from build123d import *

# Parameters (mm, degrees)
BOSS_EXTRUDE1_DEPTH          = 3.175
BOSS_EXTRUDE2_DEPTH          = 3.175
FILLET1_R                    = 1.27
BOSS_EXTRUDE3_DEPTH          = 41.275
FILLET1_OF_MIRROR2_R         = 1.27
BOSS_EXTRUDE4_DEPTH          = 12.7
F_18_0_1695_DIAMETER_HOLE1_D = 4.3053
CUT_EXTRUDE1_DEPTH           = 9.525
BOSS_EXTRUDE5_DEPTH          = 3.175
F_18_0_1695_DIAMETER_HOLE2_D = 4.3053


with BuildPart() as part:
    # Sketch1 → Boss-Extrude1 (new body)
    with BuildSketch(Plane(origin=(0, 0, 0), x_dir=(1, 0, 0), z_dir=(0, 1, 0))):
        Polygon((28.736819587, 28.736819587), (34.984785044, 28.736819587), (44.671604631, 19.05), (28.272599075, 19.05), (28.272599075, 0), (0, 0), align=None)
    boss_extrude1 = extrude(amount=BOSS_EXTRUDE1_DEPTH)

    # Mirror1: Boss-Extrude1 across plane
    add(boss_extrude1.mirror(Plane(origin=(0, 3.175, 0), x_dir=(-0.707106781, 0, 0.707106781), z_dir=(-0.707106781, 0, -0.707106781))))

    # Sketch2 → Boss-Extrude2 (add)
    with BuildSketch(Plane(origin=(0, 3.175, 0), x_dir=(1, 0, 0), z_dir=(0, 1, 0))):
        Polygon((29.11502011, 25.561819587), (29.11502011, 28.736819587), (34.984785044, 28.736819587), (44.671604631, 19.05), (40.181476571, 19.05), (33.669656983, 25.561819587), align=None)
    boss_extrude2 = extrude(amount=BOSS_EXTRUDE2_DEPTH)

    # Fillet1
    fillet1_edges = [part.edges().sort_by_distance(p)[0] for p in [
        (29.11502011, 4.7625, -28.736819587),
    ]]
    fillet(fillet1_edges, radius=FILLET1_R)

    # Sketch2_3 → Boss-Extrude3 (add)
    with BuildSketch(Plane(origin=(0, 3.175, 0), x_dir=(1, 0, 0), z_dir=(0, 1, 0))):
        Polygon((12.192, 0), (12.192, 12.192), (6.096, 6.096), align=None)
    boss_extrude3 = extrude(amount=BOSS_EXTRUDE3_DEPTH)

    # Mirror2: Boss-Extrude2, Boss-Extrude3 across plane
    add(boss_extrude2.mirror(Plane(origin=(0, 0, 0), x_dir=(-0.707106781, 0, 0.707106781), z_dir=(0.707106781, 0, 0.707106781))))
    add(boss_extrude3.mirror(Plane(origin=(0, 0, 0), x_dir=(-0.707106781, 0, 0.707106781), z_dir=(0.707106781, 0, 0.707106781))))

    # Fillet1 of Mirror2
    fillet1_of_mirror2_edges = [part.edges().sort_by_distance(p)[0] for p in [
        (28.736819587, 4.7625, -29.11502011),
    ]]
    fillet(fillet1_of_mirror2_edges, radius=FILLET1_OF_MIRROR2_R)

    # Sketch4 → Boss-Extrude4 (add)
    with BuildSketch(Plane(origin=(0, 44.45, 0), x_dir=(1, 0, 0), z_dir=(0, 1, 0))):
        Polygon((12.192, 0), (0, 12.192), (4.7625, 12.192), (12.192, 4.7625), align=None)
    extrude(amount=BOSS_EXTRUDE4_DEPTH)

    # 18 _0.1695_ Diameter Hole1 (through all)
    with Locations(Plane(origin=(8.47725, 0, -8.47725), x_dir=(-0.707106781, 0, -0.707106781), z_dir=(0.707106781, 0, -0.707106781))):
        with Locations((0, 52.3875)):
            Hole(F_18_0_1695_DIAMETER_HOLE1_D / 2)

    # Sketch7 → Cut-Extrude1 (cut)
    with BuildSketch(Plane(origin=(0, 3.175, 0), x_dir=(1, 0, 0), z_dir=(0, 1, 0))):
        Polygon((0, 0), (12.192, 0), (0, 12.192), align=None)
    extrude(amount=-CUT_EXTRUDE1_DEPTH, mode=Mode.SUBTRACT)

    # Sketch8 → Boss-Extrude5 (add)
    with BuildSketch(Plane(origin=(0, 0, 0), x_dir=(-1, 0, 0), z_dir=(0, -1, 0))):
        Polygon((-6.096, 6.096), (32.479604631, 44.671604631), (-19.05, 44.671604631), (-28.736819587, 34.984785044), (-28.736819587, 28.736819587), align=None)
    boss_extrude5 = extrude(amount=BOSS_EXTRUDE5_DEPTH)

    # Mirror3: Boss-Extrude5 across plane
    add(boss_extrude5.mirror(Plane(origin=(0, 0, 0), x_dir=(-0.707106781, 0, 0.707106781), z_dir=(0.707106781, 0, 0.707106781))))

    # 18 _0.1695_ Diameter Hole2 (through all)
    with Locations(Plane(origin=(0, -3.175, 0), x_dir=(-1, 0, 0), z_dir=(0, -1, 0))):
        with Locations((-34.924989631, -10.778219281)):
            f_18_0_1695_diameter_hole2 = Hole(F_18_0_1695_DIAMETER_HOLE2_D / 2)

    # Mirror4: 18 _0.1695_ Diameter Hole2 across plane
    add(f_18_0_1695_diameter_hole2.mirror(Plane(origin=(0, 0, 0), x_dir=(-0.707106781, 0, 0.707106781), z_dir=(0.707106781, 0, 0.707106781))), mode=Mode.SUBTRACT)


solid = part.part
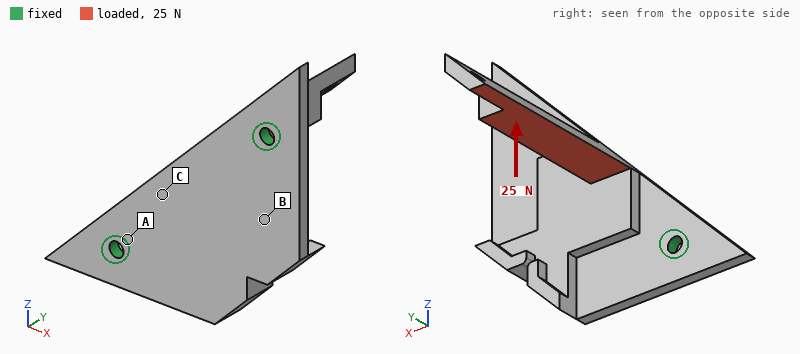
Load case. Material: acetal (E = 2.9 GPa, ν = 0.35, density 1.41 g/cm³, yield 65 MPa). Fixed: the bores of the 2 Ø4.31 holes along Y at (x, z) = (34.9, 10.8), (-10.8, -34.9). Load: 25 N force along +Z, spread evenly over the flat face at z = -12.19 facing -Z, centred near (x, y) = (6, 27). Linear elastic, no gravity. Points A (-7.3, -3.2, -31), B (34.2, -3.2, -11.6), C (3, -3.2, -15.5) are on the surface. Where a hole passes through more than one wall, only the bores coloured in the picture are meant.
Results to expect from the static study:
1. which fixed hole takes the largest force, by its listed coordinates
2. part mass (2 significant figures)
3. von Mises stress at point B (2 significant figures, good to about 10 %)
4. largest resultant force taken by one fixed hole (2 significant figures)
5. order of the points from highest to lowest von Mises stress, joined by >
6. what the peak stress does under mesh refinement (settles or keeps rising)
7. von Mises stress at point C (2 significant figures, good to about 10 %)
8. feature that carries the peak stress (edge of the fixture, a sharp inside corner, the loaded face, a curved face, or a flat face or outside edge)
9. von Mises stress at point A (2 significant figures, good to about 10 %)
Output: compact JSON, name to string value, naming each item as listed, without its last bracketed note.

{"which fixed hole takes the largest force, by its listed coordinates": "(34.9, 10.8)", "part mass": "21 g", "von Mises stress at point B": "1.0 MPa", "largest resultant force taken by one fixed hole": "22 N", "order of the points from highest to lowest von Mises stress, joined by >": "A > C > B", "what the peak stress does under mesh refinement": "keeps rising", "von Mises stress at point C": "2.4 MPa", "feature that carries the peak stress": "edge of the fixture", "von Mises stress at point A": "4.6 MPa"}
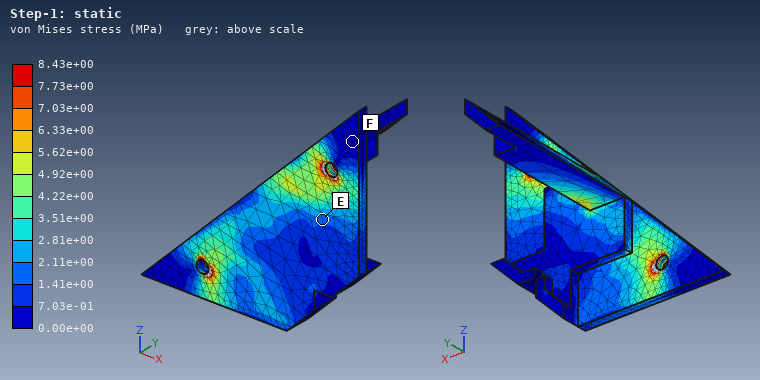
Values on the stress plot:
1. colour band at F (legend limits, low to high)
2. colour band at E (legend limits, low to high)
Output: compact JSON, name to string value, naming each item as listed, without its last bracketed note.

{"colour band at F": "0.00e+00 to 7.03e-01 MPa", "colour band at E": "1.41e+00 to 2.11e+00 MPa"}
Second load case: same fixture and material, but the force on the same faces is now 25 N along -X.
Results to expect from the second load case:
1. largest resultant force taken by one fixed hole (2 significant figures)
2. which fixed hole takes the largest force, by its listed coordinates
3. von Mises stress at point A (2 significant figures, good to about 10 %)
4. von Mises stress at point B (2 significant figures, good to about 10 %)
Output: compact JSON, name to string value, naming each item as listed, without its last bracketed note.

{"largest resultant force taken by one fixed hole": "23 N", "which fixed hole takes the largest force, by its listed coordinates": "(-10.8, -34.9)", "von Mises stress at point A": "5.7 MPa", "von Mises stress at point B": "2.1 MPa"}
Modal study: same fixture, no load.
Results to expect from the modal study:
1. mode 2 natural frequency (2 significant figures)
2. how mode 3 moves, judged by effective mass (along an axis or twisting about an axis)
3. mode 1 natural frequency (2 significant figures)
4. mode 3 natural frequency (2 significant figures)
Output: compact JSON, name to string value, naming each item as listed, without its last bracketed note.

{"mode 2 natural frequency": "660 Hz", "how mode 3 moves, judged by effective mass": "along Y", "mode 1 natural frequency": "300 Hz", "mode 3 natural frequency": "790 Hz"}
